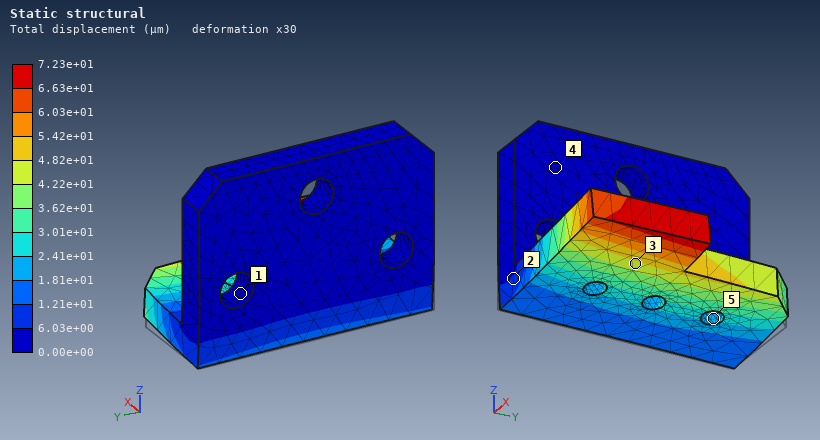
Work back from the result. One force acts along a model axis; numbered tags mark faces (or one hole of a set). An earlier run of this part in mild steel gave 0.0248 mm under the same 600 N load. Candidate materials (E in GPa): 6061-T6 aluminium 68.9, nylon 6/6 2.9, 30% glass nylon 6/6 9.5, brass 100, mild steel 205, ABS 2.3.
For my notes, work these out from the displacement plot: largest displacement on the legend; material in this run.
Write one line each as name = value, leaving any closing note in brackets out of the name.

largest displacement on the legend = 7.23e+01 µm
material in this run = 6061-T6 aluminium
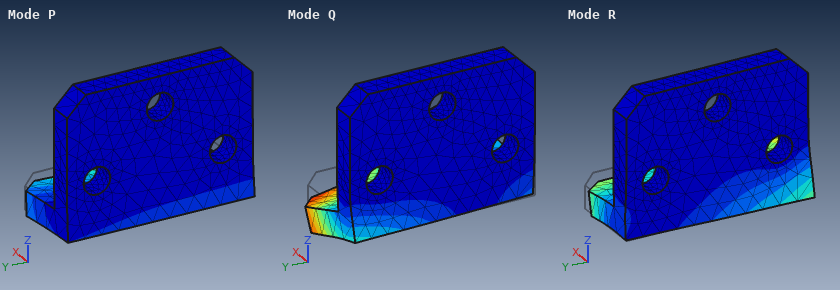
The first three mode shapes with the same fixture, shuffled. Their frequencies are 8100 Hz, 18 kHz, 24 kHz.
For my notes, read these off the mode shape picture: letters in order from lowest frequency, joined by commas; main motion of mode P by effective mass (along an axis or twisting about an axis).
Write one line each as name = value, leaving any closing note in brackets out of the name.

letters in order from lowest frequency, joined by commas = P, Q, R
main motion of mode P by effective mass = along Z
